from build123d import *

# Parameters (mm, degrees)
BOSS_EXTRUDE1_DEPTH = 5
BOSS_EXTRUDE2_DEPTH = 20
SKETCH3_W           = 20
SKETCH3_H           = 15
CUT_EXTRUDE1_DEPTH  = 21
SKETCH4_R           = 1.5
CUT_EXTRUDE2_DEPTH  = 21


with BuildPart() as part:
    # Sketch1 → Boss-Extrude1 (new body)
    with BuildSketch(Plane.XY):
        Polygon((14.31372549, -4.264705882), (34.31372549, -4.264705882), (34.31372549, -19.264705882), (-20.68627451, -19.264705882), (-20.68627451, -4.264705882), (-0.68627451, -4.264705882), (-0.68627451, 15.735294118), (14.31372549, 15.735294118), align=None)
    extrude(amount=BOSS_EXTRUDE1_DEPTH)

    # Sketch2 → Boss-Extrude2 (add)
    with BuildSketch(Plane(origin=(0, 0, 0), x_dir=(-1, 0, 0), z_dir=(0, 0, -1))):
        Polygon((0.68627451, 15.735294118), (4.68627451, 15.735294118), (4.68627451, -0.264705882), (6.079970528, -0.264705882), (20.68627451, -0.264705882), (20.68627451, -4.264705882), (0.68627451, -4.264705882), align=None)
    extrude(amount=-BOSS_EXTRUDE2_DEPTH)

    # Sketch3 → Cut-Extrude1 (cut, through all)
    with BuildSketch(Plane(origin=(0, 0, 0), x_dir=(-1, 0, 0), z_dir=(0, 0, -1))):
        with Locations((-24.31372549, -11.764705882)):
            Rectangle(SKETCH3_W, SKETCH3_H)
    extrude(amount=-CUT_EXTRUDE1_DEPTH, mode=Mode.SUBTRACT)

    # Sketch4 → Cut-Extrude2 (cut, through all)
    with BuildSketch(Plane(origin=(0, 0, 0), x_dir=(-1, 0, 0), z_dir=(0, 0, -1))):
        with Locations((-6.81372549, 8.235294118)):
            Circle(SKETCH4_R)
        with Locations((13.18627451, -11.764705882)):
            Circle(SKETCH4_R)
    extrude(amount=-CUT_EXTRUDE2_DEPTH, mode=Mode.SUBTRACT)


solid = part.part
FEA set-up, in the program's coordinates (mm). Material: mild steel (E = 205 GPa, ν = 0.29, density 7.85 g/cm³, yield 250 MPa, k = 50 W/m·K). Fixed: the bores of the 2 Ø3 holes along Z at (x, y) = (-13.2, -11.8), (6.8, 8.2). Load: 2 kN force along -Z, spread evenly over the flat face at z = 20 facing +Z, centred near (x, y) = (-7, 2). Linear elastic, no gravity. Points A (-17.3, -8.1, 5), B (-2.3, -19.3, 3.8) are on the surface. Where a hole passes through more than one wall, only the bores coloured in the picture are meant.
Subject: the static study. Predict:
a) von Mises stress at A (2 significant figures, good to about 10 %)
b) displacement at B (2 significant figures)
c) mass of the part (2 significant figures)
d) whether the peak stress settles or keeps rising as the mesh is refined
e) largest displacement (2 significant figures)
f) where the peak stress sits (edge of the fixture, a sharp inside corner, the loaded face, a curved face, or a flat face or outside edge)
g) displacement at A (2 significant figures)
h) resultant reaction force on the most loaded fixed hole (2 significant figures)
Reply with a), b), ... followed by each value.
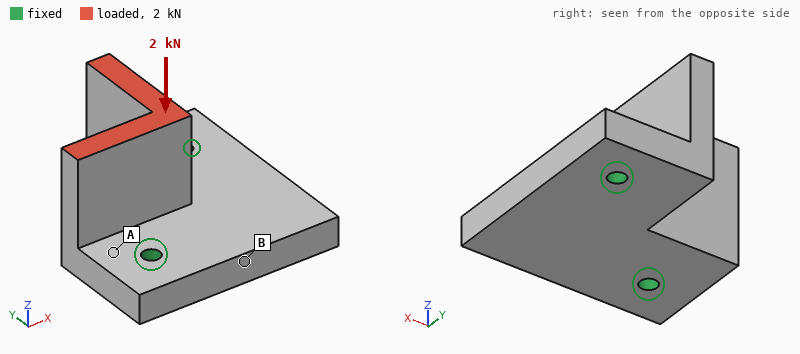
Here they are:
a) 48 MPa
b) 2.9 µm
c) 54 g
d) keeps rising
e) 18 µm
f) edge of the fixture
g) 3.8 µm
h) 1.0 kN
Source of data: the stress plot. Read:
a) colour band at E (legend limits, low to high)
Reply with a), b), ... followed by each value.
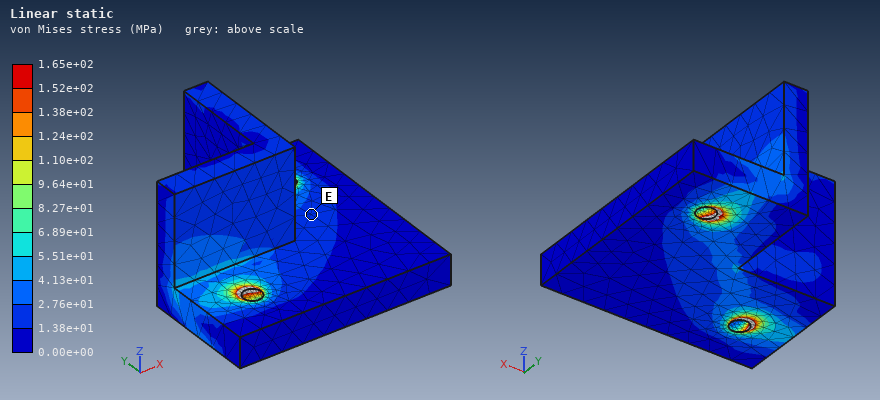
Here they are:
a) 1.38e+01 to 2.76e+01 MPa
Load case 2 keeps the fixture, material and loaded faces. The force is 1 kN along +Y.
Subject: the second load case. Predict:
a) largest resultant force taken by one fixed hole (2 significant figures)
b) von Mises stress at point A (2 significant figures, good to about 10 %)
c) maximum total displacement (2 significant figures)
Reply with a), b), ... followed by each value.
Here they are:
a) 730 N
b) 53 MPa
c) 39 µm
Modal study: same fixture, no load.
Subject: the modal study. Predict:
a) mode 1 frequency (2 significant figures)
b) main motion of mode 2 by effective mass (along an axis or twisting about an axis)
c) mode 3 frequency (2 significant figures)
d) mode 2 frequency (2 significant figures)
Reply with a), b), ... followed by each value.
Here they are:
a) 8000 Hz
b) along Z
c) 15 kHz
d) 12 kHz
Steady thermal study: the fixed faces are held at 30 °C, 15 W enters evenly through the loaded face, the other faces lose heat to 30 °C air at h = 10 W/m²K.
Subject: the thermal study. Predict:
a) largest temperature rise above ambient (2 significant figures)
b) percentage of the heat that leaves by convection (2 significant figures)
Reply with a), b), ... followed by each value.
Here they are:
a) 49 K
b) 4.0 %
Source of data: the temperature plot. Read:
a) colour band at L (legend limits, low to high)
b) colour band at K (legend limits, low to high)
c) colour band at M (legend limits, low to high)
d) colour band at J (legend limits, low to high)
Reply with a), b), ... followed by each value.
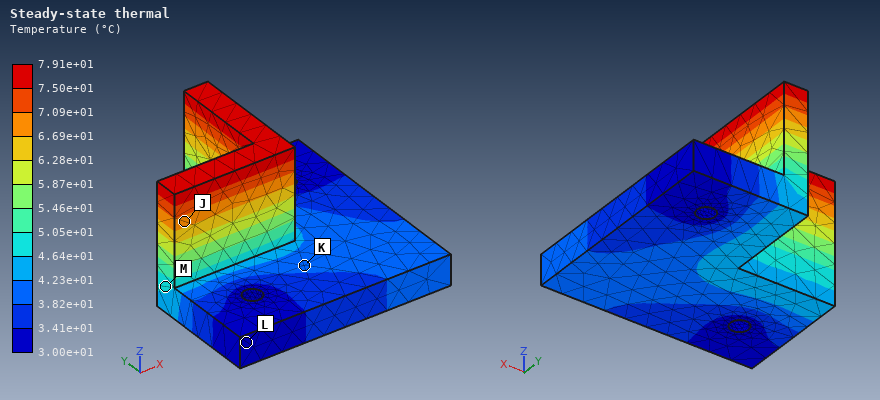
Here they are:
a) 3.00e+01 to 3.41e+01 °C
b) 3.82e+01 to 4.23e+01 °C
c) 4.64e+01 to 5.05e+01 °C
d) 6.69e+01 to 7.09e+01 °C
